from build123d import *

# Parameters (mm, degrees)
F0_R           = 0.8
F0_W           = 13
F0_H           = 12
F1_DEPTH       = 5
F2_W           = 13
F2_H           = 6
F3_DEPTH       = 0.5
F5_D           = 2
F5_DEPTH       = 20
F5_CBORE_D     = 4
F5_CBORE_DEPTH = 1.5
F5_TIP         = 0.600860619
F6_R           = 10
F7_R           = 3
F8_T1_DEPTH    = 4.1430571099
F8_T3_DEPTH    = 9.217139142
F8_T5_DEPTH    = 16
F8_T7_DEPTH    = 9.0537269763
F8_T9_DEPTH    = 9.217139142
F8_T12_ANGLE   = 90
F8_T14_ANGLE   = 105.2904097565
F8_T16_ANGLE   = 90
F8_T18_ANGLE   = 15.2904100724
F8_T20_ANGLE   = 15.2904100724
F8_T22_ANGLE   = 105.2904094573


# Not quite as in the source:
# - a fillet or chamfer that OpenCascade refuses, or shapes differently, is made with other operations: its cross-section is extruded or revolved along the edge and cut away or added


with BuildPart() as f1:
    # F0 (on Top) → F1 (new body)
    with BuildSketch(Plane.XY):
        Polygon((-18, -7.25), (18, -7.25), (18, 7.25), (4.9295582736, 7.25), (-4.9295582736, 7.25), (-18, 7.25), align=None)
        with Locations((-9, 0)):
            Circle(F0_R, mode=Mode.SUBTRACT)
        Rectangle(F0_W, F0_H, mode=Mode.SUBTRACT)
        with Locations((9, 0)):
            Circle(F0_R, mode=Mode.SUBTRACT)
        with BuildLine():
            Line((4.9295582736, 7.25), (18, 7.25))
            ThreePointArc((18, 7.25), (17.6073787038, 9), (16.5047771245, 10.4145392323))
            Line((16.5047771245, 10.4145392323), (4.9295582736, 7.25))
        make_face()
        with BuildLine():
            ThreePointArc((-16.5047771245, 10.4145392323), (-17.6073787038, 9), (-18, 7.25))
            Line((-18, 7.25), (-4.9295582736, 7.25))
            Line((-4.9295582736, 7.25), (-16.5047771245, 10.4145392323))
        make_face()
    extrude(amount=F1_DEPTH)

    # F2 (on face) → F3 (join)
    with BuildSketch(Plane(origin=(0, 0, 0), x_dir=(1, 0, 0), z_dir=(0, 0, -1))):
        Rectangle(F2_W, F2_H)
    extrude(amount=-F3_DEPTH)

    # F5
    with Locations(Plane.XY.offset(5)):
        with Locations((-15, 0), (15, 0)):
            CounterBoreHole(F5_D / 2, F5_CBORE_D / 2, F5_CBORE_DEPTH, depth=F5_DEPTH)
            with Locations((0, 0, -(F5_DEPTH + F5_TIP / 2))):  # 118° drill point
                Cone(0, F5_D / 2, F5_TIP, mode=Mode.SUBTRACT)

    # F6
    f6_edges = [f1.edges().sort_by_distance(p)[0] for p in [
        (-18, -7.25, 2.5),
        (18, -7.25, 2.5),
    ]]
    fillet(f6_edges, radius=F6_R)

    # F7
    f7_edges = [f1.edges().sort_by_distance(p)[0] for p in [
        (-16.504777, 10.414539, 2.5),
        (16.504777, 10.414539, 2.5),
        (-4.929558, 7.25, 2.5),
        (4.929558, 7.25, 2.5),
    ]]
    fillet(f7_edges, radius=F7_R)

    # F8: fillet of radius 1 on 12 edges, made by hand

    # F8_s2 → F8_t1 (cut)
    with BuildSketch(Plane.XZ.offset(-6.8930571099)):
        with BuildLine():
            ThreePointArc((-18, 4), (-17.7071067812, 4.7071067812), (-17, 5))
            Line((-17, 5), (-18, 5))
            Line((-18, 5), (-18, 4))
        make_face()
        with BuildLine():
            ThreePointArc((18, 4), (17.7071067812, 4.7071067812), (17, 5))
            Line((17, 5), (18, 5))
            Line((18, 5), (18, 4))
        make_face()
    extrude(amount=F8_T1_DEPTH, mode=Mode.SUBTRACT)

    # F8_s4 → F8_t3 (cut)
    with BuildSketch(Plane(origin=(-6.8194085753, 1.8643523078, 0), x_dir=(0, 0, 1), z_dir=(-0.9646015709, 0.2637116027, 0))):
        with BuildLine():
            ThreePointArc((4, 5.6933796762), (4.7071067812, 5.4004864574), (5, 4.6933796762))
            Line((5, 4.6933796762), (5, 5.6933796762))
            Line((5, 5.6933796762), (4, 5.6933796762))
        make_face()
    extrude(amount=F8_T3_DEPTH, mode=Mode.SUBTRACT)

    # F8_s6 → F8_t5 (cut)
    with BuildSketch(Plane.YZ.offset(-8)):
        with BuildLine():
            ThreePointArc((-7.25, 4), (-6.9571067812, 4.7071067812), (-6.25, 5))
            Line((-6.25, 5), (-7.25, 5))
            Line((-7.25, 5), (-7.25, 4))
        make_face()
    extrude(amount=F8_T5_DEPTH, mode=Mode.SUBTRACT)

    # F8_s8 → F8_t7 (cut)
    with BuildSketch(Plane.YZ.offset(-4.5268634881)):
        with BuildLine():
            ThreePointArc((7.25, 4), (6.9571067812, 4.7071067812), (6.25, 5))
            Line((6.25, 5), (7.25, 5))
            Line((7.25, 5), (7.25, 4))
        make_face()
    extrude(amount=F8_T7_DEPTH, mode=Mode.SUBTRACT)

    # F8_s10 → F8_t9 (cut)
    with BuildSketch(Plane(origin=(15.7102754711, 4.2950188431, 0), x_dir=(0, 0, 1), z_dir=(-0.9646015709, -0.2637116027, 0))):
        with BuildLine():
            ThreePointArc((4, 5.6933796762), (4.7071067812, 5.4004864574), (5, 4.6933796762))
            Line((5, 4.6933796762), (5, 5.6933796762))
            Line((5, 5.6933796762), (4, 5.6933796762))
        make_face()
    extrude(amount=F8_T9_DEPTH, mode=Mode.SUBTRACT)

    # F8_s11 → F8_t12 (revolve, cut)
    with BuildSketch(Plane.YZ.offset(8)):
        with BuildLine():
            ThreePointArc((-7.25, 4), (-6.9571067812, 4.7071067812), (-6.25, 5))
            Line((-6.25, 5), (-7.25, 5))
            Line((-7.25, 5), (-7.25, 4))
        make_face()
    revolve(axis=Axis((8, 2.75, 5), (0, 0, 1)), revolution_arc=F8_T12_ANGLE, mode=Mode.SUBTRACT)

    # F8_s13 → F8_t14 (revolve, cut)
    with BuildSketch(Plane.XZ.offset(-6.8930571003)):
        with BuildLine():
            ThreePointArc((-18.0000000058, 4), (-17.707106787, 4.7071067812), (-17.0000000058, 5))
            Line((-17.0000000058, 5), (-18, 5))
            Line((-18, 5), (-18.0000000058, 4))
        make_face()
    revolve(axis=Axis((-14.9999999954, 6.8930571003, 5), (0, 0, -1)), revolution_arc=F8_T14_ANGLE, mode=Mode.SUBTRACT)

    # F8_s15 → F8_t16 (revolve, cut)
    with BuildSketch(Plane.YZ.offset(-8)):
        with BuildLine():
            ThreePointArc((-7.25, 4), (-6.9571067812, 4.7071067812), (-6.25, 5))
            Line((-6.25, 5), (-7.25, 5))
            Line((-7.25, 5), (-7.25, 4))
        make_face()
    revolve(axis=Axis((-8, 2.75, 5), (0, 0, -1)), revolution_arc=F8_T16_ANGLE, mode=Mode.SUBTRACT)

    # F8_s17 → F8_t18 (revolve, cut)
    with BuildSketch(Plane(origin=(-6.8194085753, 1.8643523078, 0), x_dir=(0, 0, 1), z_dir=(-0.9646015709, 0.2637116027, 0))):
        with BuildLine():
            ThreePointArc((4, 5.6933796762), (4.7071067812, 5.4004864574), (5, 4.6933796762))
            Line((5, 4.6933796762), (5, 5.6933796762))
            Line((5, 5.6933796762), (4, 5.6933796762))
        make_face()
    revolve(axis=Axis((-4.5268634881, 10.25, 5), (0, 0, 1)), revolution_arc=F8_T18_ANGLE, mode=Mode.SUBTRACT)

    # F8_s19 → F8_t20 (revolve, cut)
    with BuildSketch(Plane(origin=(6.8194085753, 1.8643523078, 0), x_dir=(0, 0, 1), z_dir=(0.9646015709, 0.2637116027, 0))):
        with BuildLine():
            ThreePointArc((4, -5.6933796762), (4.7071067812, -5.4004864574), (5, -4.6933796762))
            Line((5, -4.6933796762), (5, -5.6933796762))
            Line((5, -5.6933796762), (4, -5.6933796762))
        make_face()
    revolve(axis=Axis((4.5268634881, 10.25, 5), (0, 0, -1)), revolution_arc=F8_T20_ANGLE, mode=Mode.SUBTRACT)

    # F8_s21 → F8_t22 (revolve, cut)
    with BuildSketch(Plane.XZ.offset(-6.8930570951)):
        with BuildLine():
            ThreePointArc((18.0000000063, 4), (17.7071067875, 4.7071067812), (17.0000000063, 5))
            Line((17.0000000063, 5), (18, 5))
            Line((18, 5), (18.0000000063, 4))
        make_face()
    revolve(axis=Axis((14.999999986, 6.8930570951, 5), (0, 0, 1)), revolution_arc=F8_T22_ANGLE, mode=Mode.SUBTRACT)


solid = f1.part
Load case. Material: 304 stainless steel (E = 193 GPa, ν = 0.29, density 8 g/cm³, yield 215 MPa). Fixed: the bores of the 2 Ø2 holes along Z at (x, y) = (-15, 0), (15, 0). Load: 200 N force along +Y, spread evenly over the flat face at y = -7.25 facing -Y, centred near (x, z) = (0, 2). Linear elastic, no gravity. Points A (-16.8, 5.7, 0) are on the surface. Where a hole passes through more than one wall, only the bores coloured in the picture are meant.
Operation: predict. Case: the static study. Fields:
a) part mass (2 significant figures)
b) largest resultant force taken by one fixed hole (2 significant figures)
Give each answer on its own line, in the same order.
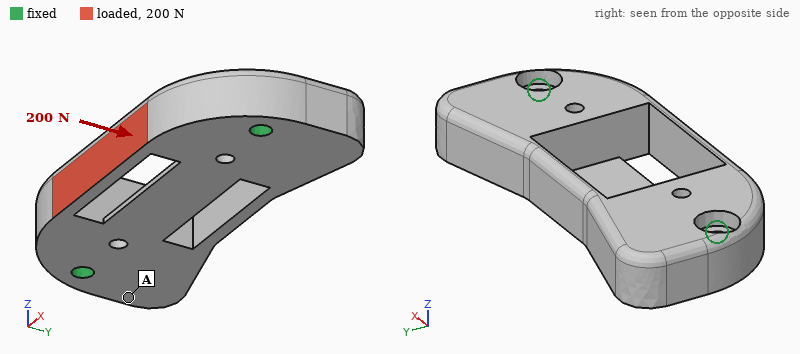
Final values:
14 g
110 N
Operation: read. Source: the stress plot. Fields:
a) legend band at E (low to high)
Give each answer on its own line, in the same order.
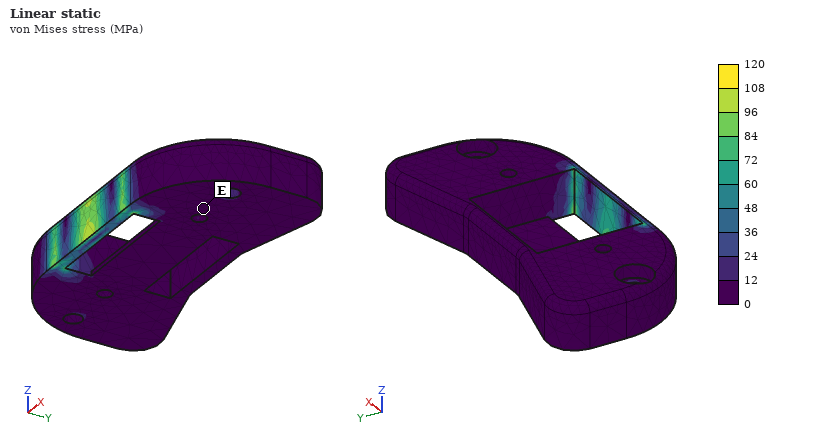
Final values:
0 to 12 MPa
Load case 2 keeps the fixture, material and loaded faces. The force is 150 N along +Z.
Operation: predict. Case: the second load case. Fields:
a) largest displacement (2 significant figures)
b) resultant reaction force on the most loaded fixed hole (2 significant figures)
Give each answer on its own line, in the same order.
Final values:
7.0 µm
75 N
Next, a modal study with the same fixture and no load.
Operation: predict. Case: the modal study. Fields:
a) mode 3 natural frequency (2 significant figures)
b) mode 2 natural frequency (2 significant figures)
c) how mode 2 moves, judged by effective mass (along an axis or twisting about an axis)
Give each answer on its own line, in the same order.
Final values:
21 kHz
19 kHz
along Z
